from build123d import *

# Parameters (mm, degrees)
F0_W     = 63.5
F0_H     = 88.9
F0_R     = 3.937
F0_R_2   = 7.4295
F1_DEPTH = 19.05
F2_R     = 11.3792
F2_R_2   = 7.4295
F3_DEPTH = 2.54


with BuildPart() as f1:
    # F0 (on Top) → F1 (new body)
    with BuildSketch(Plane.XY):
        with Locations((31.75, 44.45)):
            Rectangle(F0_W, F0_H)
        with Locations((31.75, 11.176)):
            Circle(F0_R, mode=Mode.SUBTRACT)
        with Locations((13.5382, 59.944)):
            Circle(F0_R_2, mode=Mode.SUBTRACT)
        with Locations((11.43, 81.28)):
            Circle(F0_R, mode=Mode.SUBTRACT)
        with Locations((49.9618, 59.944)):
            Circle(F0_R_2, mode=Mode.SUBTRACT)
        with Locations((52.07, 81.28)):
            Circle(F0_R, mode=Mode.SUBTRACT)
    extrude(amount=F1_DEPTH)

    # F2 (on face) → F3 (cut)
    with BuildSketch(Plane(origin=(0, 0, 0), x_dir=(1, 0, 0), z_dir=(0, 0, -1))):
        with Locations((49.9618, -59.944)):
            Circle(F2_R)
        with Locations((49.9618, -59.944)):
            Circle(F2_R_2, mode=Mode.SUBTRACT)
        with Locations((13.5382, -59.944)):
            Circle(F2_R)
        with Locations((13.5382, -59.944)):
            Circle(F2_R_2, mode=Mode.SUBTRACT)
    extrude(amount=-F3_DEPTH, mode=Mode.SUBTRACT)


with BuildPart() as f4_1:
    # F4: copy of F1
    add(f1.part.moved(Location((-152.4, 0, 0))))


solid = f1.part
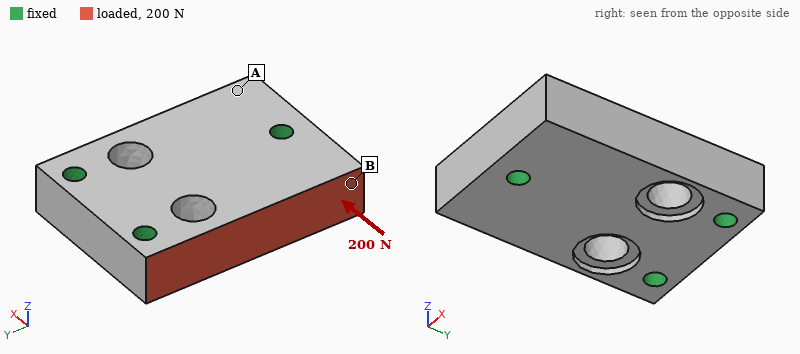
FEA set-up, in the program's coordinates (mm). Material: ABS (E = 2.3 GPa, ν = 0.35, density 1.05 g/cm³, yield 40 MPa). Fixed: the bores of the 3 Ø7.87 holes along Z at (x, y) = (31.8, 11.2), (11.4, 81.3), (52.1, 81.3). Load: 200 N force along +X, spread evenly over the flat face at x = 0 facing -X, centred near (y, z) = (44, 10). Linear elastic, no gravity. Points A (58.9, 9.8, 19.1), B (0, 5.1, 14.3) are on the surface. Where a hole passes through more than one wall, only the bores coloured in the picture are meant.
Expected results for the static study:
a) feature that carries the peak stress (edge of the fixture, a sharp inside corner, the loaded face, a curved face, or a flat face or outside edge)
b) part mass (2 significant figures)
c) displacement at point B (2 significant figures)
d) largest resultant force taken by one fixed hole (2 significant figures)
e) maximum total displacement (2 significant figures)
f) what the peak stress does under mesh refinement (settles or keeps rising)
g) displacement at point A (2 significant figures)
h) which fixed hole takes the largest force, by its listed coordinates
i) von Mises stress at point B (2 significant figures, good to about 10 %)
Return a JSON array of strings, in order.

["edge of the fixture", "100 g", "1.8 µm", "100 N", "5.6 µm", "keeps rising", "1.0 µm", "(31.8, 11.2)", "0.12 MPa"]
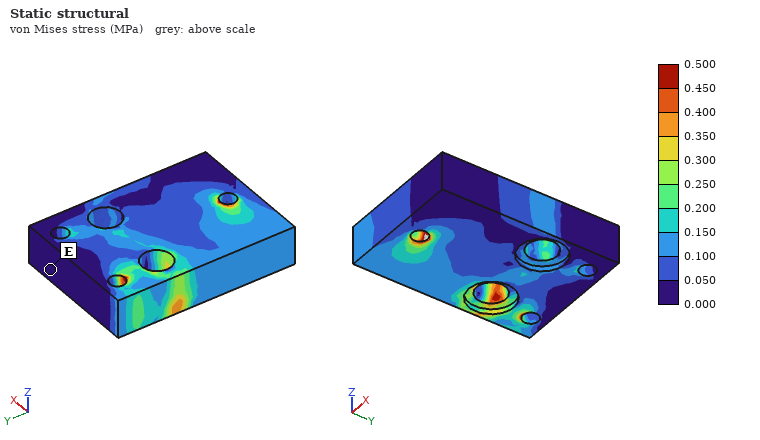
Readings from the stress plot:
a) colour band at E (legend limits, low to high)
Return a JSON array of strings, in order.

["0.000 to 0.050 MPa"]
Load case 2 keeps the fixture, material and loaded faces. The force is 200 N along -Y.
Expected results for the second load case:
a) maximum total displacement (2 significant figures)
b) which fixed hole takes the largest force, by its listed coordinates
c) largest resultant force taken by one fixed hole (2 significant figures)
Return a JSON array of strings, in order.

["9.5 µm", "(11.4, 81.3)", "110 N"]
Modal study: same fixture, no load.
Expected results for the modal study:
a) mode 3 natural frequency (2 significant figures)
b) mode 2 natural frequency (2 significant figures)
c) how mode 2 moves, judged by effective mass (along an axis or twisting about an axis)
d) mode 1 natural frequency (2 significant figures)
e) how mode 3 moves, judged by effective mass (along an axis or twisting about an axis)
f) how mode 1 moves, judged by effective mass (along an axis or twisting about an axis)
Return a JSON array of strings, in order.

["4400 Hz", "3200 Hz", "along Z", "2900 Hz", "along X", "twisting about Y"]
